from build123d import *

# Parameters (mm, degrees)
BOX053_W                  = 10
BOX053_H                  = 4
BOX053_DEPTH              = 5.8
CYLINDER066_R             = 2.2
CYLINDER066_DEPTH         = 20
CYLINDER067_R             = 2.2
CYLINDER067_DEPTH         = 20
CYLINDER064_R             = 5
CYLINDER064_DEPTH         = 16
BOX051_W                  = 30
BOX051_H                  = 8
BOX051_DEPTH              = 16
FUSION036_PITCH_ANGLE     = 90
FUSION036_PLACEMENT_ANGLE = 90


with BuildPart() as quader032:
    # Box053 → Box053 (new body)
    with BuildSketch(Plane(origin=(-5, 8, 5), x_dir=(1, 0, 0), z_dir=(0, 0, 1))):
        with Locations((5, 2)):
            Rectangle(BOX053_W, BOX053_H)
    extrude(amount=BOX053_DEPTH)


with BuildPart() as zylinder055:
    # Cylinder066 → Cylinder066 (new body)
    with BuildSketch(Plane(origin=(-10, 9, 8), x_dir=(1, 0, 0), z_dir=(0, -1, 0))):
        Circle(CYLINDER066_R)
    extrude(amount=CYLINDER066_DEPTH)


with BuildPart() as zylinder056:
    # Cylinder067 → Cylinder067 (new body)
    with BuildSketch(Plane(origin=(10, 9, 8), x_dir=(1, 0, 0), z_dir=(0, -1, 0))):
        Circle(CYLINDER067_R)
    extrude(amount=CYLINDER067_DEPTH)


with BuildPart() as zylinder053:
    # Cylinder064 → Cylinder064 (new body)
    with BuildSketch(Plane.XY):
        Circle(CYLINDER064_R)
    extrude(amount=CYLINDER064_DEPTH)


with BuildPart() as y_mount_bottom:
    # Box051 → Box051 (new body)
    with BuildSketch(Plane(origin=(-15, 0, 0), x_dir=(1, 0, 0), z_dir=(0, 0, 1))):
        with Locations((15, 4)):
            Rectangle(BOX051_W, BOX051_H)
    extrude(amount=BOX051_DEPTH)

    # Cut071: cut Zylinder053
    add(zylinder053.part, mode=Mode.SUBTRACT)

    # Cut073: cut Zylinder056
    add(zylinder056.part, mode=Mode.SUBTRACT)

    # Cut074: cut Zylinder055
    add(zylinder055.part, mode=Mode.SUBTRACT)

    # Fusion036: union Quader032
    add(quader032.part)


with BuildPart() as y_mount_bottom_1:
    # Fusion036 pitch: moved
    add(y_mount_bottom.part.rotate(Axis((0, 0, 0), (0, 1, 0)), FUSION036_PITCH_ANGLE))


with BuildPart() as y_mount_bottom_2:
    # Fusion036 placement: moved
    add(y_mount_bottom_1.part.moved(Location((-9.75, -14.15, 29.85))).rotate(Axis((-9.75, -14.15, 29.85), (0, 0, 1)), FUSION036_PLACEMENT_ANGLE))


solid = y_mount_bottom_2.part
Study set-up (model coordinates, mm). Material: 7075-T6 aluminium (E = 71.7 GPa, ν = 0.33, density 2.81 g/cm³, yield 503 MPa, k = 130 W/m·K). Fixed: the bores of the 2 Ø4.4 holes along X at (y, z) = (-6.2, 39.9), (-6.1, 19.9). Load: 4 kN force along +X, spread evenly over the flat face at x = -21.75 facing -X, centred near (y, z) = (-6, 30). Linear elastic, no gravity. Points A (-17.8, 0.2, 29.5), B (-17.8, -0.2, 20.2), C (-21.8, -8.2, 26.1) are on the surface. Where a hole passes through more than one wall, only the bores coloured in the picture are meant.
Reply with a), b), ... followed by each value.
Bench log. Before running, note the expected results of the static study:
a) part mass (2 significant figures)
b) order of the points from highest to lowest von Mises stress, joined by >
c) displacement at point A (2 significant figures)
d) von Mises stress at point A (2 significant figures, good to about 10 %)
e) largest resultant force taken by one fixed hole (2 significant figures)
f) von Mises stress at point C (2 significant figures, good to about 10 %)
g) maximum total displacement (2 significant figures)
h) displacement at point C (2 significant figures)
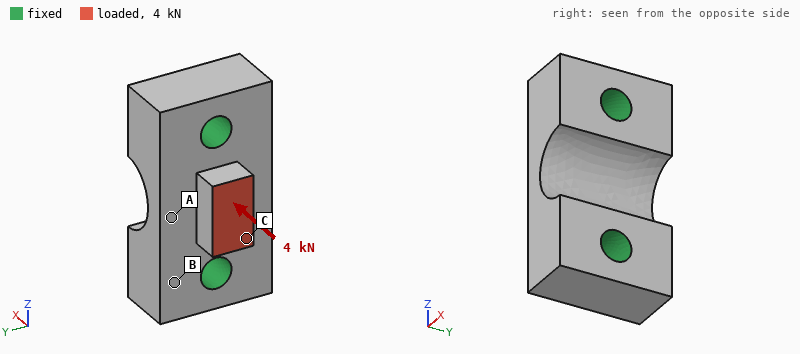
a) 9.0 g
b) C > A > B
c) 6.8 µm
d) 32 MPa
e) 2.3 kN
f) 69 MPa
g) 14 µm
h) 13 µm
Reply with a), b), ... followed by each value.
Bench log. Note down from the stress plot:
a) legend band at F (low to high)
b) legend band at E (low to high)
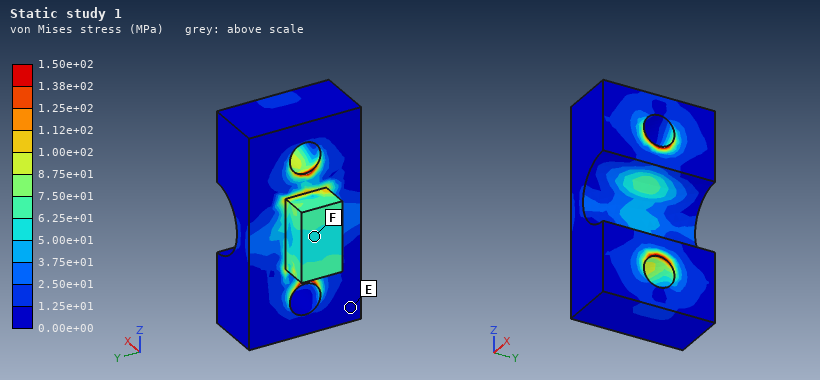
a) 5.00e+01 to 6.25e+01 MPa
b) 0.00e+00 to 1.25e+01 MPa
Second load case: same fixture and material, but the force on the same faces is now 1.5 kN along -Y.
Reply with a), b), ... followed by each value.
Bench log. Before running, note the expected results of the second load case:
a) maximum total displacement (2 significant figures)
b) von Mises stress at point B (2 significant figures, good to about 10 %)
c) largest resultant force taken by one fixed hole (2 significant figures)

a) 25 µm
b) 10 MPa
c) 750 N
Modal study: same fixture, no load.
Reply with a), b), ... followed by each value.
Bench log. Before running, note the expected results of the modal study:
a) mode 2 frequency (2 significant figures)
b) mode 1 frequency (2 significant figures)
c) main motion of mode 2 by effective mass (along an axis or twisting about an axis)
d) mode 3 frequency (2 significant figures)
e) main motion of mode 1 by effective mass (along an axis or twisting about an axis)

a) 62 kHz
b) 49 kHz
c) along X
d) 71 kHz
e) along Y
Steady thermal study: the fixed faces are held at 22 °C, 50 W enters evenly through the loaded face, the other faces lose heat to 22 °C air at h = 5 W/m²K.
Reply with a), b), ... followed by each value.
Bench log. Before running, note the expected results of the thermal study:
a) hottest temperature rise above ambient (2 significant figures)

a) 50 K
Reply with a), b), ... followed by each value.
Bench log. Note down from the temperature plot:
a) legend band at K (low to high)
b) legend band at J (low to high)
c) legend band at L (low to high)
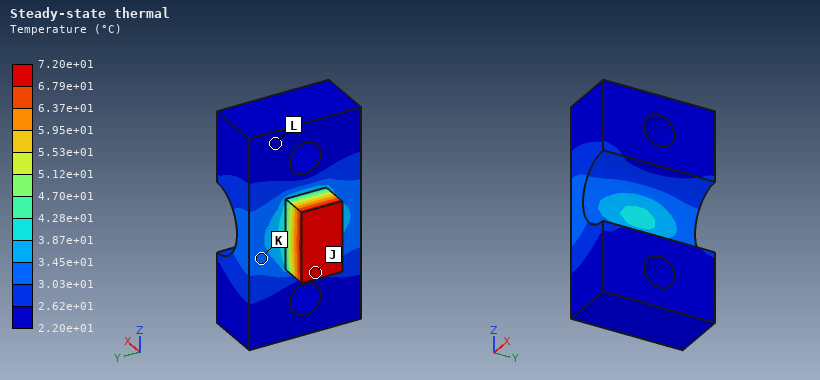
a) 3.03e+01 to 3.45e+01 °C
b) 6.79e+01 to 7.20e+01 °C
c) 2.20e+01 to 2.62e+01 °C
